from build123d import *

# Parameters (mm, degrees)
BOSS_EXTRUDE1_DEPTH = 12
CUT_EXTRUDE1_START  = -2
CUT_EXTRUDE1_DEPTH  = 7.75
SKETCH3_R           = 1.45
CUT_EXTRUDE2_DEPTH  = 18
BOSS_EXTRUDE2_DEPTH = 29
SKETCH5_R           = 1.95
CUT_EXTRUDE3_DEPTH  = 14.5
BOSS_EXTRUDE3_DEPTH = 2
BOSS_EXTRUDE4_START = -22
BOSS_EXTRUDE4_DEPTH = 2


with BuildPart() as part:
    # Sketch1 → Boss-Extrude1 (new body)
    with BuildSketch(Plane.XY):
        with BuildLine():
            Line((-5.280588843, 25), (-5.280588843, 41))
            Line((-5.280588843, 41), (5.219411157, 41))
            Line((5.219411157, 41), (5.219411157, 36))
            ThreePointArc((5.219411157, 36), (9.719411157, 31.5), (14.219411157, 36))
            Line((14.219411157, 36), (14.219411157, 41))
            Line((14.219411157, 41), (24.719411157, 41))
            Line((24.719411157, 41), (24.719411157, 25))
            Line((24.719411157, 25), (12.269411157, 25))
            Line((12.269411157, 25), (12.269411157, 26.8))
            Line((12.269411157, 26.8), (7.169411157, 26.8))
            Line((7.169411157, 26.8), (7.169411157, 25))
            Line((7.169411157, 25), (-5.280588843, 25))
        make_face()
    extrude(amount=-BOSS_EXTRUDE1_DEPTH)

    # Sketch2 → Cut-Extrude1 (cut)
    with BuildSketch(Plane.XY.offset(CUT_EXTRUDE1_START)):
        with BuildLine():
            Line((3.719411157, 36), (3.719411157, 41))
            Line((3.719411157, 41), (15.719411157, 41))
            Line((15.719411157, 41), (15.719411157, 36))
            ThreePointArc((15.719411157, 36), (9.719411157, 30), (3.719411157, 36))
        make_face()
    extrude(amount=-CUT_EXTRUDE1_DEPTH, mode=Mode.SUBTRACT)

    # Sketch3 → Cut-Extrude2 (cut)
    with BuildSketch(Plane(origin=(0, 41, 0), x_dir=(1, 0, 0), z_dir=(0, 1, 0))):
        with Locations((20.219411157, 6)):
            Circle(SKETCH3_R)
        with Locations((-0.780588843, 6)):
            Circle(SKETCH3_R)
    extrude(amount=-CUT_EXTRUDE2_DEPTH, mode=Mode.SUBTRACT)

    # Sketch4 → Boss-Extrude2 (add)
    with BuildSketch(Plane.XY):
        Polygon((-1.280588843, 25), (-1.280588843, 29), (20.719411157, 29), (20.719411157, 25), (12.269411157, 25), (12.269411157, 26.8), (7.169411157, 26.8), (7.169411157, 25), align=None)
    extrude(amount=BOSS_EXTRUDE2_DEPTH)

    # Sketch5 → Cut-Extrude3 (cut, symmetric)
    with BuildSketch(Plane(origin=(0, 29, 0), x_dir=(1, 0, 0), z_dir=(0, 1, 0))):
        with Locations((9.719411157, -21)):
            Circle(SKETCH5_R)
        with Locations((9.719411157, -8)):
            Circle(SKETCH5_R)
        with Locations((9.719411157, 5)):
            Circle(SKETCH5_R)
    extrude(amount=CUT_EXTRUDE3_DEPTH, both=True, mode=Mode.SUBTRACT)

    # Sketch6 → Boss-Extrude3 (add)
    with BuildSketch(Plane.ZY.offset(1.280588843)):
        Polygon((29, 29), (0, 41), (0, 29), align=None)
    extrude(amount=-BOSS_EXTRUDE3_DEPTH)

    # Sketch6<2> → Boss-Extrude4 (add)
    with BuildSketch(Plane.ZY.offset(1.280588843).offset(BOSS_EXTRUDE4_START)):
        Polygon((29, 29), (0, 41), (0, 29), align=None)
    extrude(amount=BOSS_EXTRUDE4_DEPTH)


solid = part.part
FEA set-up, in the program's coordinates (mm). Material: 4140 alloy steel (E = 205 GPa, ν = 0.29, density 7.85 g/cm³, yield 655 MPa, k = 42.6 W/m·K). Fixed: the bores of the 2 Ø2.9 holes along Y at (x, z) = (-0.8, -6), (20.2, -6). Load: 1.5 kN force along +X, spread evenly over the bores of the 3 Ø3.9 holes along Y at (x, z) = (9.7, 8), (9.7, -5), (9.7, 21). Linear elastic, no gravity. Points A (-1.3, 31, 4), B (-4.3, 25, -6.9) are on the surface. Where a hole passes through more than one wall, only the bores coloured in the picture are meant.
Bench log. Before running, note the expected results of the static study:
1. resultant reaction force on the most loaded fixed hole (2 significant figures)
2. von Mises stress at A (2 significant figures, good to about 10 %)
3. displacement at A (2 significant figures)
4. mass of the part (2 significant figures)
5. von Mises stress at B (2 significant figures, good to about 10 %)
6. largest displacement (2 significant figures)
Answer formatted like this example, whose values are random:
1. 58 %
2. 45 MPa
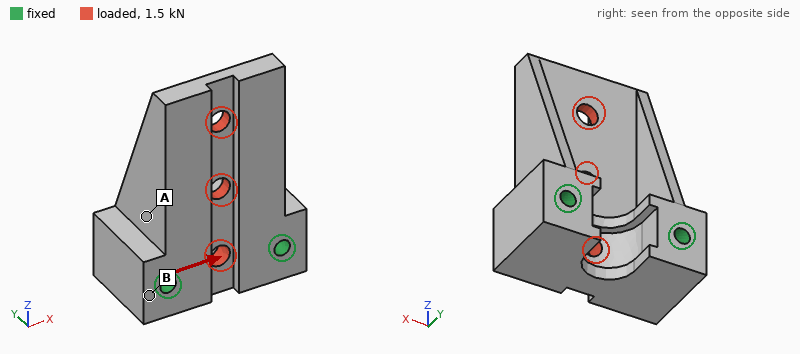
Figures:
1. 1.1 kN
2. 18 MPa
3. 1.7 µm
4. 56 g
5. 7.4 MPa
6. 9.0 µm
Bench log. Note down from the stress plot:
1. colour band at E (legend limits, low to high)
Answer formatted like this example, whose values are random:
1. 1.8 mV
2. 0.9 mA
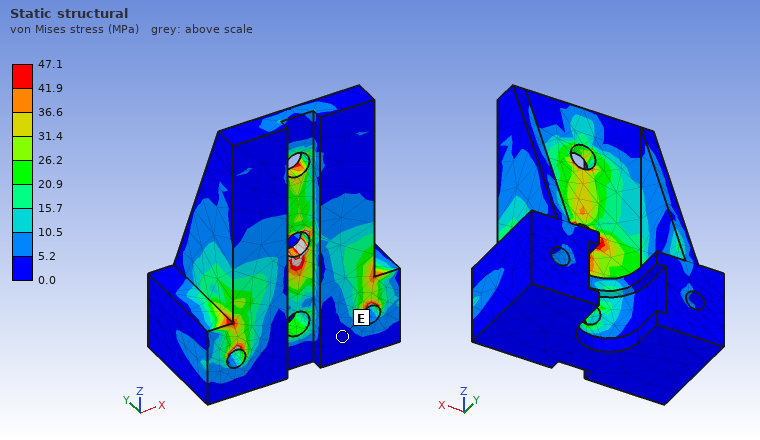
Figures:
1. 0.0 to 5.2 MPa
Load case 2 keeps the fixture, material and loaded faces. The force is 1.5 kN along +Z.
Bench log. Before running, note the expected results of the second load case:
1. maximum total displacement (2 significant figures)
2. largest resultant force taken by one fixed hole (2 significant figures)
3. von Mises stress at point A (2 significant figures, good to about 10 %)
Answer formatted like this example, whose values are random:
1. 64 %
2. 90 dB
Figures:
1. 2.5 µm
2. 760 N
3. 8.5 MPa
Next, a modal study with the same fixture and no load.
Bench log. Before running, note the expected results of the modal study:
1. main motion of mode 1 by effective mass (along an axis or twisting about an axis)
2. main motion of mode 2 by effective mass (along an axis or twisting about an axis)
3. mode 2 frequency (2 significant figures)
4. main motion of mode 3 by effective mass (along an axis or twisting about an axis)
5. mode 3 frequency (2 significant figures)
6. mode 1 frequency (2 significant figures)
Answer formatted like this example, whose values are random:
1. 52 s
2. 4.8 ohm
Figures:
1. along Y
2. along X
3. 12 kHz
4. along X
5. 17 kHz
6. 8800 Hz
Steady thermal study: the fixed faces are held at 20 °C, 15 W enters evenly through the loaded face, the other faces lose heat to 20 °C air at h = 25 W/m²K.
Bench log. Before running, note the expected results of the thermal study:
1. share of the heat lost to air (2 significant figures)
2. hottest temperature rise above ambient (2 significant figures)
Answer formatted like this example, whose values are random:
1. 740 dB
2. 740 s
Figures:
1. 9.6 %
2. 40 K
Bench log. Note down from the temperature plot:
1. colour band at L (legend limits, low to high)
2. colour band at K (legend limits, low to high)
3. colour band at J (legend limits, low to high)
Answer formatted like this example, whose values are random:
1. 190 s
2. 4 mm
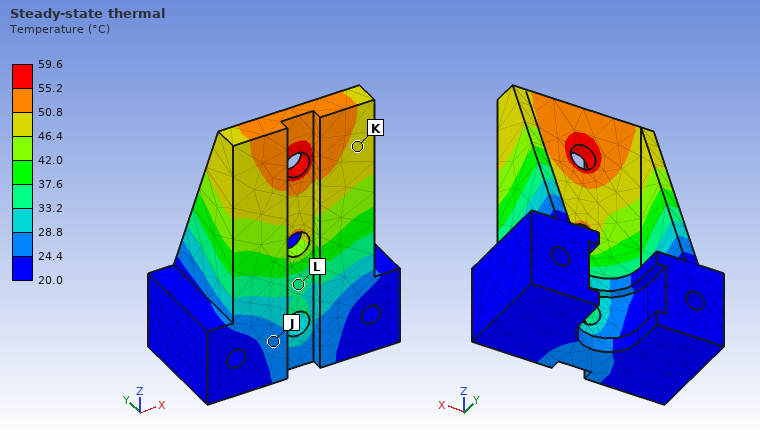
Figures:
1. 33.2 to 37.6 °C
2. 46.4 to 50.8 °C
3. 24.4 to 28.8 °C
